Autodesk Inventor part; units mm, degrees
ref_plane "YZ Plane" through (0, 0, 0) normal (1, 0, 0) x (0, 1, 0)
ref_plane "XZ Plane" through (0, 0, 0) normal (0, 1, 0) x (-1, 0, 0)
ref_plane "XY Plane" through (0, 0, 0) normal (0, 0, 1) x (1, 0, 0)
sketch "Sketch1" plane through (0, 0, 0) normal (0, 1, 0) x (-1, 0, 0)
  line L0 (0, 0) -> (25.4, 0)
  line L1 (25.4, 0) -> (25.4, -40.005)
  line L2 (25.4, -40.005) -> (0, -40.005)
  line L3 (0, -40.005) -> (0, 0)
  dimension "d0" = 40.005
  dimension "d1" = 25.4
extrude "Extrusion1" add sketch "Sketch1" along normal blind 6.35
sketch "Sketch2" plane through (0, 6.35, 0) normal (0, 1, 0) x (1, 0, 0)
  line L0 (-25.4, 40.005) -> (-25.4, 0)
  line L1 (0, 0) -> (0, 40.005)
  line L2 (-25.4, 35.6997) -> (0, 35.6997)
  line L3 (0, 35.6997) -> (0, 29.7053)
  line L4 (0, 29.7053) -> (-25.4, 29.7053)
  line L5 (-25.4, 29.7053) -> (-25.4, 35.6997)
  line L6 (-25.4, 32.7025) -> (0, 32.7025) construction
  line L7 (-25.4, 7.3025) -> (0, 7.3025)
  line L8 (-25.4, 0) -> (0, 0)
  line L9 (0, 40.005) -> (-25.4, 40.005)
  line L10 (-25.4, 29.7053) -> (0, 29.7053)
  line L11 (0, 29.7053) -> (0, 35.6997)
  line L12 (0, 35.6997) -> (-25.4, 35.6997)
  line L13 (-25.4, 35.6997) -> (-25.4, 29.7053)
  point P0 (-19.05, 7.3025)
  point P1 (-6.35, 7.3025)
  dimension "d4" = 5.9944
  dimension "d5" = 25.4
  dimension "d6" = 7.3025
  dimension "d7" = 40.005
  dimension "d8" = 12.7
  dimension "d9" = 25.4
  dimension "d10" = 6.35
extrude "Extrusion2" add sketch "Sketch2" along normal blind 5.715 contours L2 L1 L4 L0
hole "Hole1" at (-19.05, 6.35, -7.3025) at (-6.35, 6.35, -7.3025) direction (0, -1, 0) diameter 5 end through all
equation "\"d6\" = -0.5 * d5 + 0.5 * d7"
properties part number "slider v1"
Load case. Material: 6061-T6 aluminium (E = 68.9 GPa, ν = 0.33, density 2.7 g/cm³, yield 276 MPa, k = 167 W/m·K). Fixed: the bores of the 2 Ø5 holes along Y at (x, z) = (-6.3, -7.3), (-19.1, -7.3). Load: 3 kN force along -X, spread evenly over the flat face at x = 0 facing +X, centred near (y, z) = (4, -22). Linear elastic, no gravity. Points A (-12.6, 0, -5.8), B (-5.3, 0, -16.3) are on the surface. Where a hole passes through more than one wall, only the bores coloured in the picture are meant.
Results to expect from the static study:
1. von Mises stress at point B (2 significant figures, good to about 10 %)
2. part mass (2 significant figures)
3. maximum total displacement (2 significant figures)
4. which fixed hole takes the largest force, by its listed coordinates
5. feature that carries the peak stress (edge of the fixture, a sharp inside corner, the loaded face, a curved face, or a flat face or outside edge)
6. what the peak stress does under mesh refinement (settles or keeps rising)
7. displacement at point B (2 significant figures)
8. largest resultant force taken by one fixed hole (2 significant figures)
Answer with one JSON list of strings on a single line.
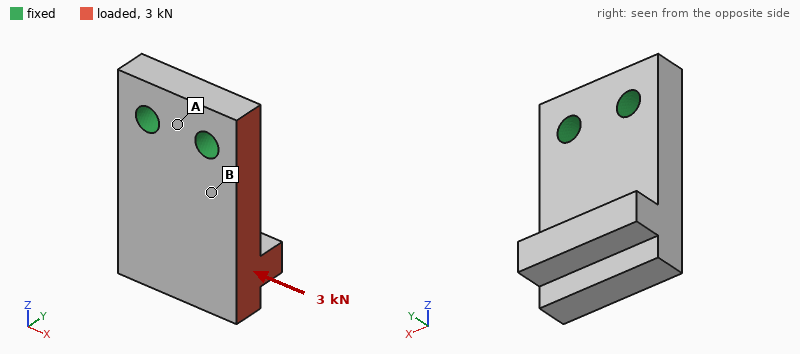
["34 MPa", "19 g", "42 µm", "(-6.3, -7.3)", "edge of the fixture", "keeps rising", "9.2 µm", "3.1 kN"]
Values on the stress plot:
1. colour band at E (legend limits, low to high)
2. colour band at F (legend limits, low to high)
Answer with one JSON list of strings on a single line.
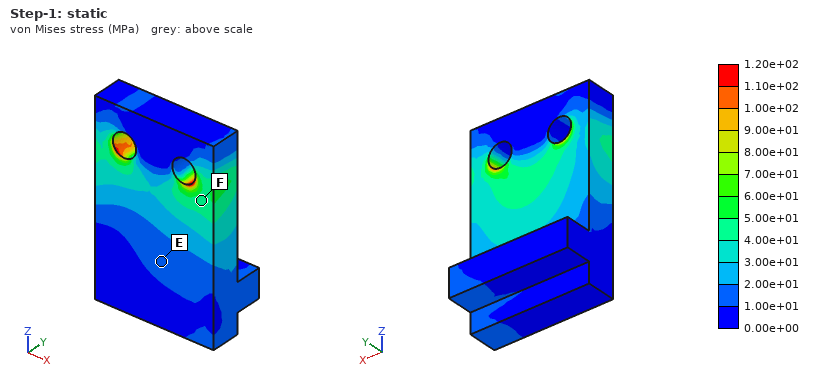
["1.00e+01 to 2.00e+01 MPa", "4.00e+01 to 5.00e+01 MPa"]
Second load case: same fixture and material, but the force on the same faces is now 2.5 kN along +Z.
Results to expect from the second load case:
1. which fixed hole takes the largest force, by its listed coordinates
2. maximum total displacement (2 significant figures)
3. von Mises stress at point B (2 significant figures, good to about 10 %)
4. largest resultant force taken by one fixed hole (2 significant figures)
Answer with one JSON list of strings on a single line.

["(-6.3, -7.3)", "40 µm", "23 MPa", "3.2 kN"]
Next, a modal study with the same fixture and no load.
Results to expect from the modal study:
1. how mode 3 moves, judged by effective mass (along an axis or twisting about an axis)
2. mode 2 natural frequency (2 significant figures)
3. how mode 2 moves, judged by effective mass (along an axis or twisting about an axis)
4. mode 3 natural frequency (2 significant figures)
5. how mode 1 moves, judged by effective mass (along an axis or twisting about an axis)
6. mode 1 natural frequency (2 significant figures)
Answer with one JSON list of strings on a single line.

["along X", "11 kHz", "along X", "13 kHz", "along Y", "4400 Hz"]
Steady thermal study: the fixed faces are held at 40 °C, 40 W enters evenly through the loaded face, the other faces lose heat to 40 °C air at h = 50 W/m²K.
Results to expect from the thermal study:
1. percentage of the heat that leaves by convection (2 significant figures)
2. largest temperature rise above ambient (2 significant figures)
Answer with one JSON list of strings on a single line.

["4.1 %", "26 K"]
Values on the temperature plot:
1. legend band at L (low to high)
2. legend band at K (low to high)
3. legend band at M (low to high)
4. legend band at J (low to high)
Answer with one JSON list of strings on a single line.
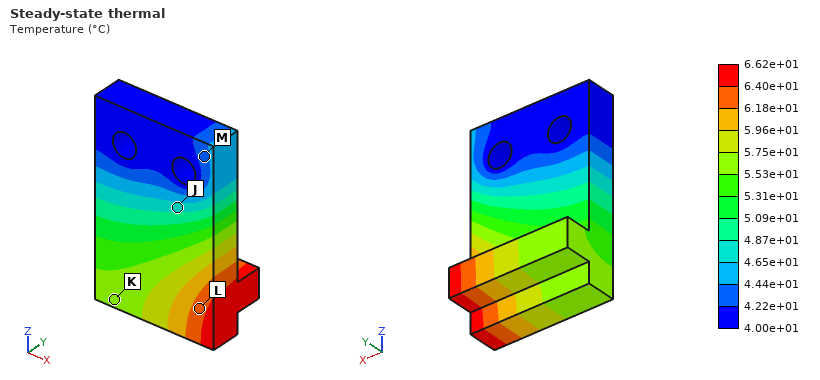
["6.18e+01 to 6.40e+01 °C", "5.53e+01 to 5.75e+01 °C", "4.22e+01 to 4.44e+01 °C", "4.65e+01 to 4.87e+01 °C"]
